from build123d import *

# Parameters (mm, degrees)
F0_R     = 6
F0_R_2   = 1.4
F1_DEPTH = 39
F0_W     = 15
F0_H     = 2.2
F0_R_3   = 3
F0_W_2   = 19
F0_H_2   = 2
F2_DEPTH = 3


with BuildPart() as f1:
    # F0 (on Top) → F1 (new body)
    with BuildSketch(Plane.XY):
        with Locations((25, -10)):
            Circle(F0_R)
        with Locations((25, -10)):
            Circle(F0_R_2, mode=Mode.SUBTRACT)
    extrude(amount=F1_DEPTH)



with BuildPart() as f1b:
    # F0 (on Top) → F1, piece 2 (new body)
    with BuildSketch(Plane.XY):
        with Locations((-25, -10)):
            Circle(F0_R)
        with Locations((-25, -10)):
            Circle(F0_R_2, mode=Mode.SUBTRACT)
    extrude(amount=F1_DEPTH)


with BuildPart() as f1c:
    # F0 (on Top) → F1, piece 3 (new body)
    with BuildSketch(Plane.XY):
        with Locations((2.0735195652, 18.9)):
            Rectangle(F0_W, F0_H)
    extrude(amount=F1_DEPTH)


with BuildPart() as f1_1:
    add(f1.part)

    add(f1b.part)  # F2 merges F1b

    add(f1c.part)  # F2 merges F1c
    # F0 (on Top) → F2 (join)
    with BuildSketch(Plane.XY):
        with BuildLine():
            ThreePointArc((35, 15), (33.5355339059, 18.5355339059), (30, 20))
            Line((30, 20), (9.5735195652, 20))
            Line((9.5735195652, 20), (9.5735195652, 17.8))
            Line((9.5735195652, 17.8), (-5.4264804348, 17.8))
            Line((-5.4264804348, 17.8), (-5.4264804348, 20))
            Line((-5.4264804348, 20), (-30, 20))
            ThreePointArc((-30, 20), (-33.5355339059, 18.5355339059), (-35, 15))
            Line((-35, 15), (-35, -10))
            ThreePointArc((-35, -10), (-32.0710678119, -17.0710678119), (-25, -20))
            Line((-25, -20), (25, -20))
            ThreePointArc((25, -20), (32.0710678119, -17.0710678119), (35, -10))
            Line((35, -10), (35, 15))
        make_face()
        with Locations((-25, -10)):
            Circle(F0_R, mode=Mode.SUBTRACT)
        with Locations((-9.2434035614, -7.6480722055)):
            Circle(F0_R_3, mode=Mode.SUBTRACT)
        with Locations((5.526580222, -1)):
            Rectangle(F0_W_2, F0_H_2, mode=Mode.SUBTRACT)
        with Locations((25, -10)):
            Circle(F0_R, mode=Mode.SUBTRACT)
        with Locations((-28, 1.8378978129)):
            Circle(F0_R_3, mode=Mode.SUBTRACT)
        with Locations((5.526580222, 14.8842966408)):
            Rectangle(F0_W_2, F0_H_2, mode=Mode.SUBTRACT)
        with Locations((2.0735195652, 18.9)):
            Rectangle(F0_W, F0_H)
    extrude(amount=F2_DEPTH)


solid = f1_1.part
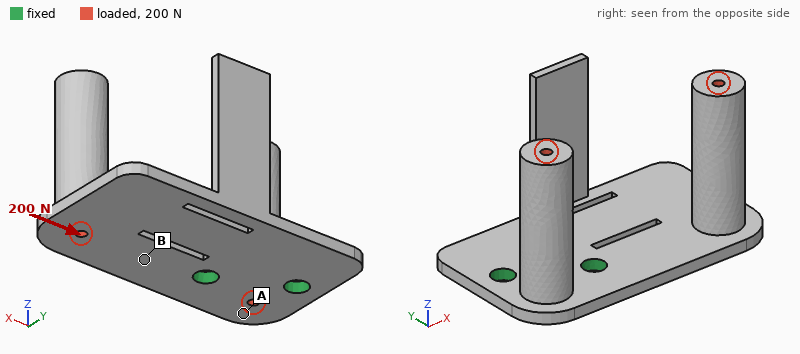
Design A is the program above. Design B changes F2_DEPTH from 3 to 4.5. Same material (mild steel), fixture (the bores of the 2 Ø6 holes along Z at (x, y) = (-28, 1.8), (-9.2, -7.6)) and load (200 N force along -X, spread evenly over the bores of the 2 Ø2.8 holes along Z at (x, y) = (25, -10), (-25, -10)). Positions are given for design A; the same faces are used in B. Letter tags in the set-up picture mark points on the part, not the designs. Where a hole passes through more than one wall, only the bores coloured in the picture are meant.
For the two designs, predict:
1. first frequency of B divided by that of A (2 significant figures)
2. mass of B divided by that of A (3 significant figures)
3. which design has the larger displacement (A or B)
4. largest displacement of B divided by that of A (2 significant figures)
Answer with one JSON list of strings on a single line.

["1.7", "1.21", "A", "0.30"]
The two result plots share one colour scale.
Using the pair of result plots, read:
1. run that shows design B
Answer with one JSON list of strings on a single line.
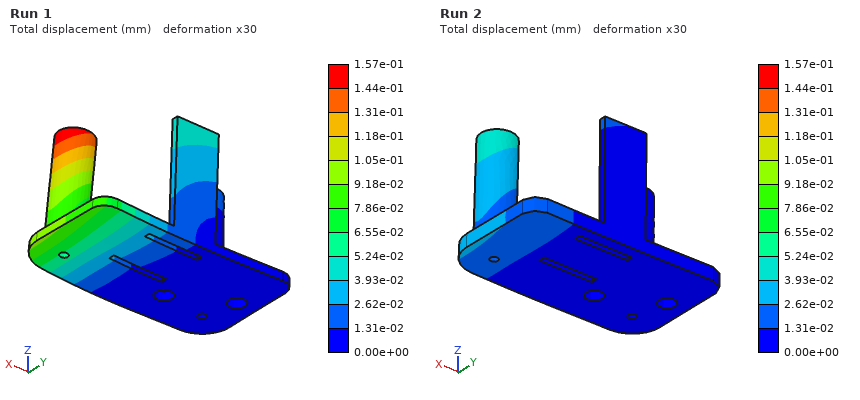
["Run 2"]
